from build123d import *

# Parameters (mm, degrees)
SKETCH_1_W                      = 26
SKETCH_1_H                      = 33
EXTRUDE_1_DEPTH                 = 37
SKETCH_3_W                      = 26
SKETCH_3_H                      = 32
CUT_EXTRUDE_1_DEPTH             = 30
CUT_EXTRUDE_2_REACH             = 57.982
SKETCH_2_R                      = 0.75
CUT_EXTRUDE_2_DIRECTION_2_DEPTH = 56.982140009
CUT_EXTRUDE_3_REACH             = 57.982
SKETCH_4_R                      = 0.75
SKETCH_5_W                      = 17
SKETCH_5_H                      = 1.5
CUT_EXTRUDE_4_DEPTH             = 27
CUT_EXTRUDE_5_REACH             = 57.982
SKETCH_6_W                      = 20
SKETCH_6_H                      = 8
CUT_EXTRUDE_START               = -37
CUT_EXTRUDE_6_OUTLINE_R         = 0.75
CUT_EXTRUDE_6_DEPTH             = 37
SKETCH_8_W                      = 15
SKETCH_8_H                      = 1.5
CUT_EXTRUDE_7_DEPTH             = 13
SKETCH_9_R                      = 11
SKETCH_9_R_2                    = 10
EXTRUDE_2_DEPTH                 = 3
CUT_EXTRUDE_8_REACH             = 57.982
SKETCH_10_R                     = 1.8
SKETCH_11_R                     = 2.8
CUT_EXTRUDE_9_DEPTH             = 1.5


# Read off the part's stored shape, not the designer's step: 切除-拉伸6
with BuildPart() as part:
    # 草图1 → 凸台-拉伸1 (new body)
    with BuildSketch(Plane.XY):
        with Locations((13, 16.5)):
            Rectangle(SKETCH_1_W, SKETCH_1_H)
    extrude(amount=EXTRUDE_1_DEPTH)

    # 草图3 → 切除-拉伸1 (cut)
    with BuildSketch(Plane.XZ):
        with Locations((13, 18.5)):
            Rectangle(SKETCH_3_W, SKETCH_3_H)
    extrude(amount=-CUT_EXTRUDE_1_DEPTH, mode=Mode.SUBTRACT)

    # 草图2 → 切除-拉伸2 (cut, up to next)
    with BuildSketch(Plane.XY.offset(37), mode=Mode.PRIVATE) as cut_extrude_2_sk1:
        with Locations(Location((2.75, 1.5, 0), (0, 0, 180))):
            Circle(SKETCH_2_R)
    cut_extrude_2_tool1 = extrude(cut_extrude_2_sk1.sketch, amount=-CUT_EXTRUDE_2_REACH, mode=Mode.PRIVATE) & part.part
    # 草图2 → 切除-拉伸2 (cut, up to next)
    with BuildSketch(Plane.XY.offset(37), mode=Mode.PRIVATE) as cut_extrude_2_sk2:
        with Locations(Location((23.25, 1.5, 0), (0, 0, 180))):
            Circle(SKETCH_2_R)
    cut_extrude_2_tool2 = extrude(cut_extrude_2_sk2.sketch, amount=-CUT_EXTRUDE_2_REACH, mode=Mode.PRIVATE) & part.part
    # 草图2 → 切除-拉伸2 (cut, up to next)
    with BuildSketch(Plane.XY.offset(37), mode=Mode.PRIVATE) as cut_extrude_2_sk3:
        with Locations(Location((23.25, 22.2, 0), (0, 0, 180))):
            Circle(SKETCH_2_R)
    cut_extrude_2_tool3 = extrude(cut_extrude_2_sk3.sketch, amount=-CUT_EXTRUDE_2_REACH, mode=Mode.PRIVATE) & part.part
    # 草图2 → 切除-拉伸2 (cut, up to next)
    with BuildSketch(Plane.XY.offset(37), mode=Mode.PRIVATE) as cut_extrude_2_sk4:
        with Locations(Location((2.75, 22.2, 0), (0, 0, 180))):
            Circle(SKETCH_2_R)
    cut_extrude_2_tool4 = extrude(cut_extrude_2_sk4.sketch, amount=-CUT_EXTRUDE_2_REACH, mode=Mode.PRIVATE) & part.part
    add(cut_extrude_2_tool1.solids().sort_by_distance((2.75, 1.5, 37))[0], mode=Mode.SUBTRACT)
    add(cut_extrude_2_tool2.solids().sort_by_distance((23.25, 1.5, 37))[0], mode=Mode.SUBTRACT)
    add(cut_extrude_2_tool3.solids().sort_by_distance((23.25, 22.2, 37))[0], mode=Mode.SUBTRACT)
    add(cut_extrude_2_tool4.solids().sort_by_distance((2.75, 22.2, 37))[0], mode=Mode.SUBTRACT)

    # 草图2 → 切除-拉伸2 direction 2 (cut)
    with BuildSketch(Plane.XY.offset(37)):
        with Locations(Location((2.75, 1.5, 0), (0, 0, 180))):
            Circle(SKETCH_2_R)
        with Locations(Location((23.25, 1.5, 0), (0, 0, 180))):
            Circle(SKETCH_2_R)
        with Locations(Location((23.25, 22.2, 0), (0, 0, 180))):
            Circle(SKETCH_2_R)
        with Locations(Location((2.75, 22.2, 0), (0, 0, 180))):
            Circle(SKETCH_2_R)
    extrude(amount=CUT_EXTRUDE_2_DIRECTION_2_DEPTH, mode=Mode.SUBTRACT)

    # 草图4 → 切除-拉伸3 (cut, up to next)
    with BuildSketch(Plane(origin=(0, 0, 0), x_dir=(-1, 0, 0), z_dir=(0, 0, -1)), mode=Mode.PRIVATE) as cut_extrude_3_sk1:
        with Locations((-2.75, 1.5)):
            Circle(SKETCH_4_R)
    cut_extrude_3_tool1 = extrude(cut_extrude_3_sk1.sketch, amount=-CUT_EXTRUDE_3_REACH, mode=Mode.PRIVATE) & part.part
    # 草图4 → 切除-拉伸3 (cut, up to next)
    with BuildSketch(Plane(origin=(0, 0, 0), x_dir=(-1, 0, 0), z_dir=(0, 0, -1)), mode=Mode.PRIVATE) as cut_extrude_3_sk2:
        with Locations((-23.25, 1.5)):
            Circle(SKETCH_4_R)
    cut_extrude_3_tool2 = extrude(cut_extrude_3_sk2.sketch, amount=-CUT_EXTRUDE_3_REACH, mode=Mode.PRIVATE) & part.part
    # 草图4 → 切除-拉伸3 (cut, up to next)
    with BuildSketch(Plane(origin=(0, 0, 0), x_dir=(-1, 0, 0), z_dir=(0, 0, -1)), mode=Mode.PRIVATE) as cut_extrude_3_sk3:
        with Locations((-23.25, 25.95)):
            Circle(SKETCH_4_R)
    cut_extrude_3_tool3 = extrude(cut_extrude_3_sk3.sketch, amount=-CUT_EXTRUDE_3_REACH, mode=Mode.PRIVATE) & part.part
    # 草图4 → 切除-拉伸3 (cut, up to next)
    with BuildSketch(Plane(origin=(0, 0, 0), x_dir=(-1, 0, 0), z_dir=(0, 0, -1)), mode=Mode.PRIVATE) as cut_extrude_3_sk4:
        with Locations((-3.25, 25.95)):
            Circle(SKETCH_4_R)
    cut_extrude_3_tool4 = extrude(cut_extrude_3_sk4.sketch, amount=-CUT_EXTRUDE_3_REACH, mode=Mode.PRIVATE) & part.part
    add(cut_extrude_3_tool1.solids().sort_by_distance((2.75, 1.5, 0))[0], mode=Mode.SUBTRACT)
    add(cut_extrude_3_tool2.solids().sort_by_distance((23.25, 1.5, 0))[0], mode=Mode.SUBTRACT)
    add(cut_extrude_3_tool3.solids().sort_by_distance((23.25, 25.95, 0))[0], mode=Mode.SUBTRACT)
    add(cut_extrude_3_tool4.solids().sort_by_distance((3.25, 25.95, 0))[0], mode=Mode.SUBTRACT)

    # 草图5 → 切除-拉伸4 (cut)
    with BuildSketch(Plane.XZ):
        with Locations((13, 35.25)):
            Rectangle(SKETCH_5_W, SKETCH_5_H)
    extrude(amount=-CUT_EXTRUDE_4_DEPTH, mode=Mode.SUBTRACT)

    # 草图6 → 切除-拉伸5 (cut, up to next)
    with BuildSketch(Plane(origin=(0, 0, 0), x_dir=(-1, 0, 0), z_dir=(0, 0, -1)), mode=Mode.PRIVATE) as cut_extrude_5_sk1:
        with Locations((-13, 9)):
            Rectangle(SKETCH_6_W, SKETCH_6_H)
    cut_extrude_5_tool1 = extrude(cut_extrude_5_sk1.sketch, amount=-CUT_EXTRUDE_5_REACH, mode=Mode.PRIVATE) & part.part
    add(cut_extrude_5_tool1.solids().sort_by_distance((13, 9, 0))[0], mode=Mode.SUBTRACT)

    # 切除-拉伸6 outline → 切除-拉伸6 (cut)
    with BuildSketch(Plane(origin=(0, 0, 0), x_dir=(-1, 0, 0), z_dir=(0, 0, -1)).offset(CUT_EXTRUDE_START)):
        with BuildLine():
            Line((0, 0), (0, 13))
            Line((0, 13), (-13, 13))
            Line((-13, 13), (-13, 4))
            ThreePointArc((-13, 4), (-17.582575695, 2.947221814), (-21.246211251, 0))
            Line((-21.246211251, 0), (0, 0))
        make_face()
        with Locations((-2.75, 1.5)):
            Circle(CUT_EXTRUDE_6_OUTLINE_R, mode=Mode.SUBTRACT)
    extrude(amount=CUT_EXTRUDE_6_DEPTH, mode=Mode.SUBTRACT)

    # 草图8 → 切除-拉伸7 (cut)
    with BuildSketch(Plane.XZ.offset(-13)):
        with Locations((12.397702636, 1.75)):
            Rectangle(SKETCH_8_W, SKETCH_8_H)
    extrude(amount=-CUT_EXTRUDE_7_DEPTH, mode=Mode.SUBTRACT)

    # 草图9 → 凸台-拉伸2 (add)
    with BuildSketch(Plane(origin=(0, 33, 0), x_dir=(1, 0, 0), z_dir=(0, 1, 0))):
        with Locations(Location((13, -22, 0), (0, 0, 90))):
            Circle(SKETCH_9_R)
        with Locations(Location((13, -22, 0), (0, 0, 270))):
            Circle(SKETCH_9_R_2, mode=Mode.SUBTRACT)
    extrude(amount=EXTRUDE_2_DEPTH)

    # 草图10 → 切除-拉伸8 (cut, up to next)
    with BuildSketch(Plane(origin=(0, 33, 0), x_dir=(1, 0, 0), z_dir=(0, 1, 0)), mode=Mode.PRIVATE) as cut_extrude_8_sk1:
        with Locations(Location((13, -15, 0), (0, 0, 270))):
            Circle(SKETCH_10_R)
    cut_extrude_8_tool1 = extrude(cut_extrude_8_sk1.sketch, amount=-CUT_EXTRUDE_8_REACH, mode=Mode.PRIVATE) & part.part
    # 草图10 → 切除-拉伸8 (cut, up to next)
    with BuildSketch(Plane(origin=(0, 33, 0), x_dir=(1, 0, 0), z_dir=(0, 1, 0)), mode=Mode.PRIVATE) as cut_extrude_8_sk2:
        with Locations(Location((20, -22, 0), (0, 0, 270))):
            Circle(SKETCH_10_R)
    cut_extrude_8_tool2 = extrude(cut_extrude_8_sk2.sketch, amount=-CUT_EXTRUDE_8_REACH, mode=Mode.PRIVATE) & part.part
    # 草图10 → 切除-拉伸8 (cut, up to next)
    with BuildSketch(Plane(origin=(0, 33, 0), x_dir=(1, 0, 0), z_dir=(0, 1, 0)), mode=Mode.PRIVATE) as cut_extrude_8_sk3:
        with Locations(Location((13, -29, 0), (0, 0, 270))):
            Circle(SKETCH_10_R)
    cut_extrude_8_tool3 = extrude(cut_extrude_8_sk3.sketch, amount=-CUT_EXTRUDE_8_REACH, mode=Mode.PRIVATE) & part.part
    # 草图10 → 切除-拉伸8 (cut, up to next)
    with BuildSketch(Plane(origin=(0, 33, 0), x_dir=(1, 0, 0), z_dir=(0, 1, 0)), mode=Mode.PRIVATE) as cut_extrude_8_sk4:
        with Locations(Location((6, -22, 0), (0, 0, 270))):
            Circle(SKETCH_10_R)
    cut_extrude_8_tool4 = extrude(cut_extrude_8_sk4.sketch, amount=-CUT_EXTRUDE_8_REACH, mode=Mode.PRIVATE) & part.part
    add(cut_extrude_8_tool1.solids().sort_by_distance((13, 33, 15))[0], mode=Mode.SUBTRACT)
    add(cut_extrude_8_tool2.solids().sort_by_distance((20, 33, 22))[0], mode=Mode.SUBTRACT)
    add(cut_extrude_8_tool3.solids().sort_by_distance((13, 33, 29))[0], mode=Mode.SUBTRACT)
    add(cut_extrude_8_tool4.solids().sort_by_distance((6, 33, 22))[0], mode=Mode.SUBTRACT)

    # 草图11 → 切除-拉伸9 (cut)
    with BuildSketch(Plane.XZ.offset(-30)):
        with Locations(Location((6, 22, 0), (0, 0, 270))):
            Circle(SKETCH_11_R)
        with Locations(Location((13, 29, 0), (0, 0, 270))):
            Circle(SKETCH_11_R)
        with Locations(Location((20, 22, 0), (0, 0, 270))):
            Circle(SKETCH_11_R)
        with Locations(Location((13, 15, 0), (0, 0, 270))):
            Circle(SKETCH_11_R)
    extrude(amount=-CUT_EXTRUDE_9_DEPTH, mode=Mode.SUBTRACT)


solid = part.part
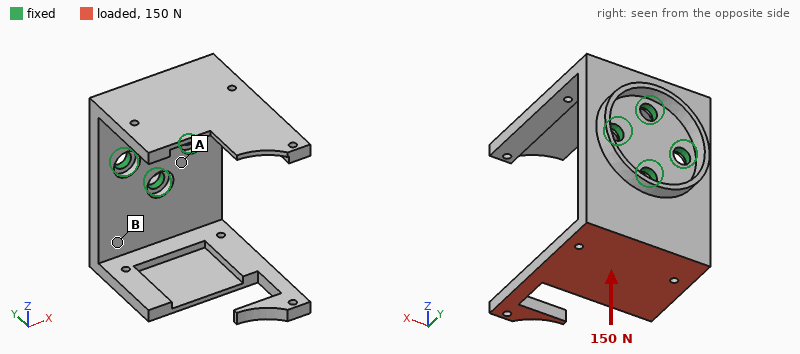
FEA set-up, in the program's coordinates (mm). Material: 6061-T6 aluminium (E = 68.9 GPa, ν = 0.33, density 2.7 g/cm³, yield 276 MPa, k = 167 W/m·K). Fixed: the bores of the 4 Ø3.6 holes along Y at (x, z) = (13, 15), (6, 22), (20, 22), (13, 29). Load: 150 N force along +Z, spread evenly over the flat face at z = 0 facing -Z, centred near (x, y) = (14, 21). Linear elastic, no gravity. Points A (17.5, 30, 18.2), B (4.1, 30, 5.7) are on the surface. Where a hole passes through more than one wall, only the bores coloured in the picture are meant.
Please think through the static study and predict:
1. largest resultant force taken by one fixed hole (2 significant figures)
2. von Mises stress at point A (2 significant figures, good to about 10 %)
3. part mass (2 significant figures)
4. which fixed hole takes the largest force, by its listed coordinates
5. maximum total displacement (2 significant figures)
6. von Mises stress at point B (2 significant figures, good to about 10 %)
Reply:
170 N
17 MPa
13 g
(13, 15)
0.47 mm
37 MPa
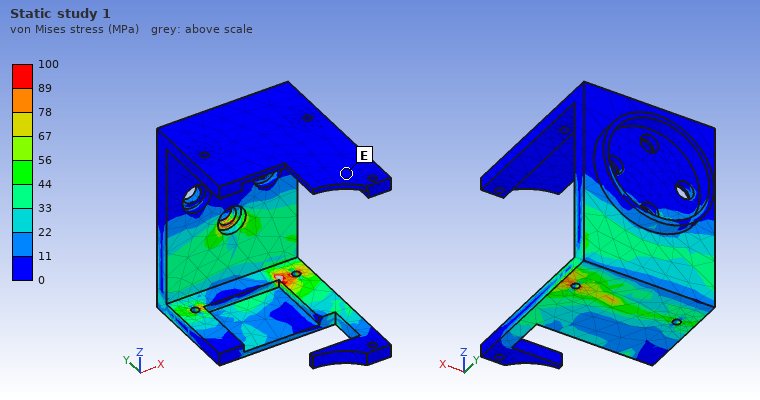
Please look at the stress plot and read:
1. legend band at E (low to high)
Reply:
0 to 11 MPa
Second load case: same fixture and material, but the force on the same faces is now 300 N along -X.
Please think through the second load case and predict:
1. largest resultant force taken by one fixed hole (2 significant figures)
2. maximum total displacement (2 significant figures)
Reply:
370 N
0.31 mm
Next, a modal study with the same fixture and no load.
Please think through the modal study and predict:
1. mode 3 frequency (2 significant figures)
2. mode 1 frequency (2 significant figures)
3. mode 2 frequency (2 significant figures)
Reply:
3400 Hz
2000 Hz
2100 Hz
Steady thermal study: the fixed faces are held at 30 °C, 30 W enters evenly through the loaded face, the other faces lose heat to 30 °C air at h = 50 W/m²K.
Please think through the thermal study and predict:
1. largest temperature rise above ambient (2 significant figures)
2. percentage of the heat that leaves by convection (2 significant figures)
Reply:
88 K
12 %
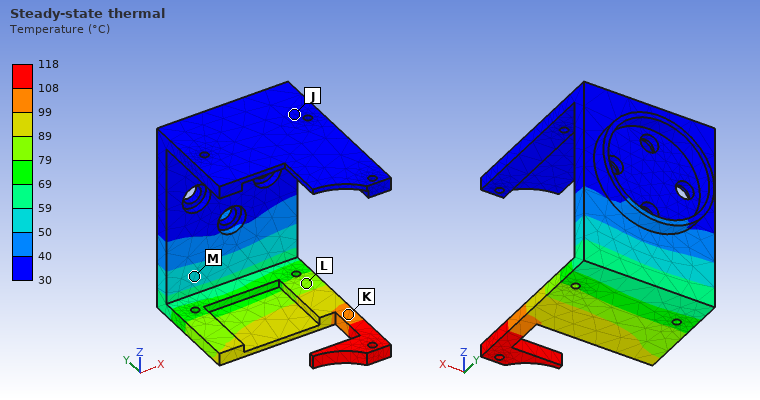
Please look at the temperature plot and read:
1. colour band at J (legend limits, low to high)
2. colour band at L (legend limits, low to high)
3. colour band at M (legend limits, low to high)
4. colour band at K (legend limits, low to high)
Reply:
30 to 40 °C
79 to 89 °C
50 to 59 °C
99 to 108 °C
